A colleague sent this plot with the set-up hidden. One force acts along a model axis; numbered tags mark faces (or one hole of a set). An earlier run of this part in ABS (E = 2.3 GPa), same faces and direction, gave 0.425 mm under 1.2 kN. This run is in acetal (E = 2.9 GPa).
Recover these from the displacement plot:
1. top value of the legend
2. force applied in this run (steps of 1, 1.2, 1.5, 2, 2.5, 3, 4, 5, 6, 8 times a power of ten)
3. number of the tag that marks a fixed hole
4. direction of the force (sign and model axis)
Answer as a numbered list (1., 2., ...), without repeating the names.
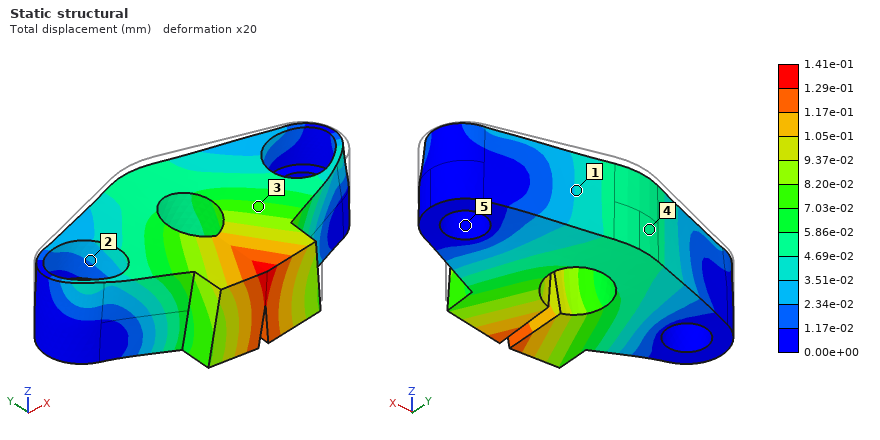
1. 1.41e-01 mm
2. 500 N
3. 5
4. -Z
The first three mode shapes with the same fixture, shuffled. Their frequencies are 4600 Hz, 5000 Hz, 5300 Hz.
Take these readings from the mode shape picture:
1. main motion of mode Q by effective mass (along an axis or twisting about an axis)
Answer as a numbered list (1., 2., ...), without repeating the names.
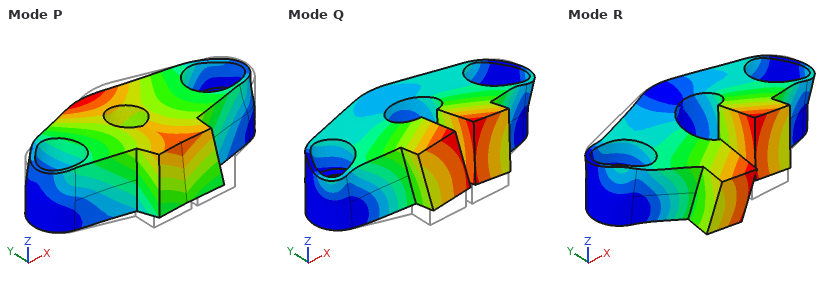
1. along Z
